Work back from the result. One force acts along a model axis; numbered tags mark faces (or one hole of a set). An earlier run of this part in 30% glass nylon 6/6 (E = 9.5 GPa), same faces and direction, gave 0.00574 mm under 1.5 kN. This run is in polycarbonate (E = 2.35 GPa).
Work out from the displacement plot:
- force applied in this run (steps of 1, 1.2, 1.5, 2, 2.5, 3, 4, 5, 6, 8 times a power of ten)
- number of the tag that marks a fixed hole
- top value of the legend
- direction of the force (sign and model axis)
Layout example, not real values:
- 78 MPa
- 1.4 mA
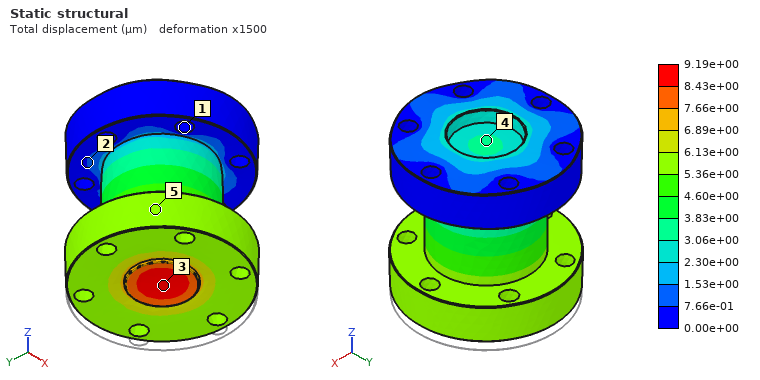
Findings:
- 600 N
- 1
- 9.19e+00 µm
- +Z
